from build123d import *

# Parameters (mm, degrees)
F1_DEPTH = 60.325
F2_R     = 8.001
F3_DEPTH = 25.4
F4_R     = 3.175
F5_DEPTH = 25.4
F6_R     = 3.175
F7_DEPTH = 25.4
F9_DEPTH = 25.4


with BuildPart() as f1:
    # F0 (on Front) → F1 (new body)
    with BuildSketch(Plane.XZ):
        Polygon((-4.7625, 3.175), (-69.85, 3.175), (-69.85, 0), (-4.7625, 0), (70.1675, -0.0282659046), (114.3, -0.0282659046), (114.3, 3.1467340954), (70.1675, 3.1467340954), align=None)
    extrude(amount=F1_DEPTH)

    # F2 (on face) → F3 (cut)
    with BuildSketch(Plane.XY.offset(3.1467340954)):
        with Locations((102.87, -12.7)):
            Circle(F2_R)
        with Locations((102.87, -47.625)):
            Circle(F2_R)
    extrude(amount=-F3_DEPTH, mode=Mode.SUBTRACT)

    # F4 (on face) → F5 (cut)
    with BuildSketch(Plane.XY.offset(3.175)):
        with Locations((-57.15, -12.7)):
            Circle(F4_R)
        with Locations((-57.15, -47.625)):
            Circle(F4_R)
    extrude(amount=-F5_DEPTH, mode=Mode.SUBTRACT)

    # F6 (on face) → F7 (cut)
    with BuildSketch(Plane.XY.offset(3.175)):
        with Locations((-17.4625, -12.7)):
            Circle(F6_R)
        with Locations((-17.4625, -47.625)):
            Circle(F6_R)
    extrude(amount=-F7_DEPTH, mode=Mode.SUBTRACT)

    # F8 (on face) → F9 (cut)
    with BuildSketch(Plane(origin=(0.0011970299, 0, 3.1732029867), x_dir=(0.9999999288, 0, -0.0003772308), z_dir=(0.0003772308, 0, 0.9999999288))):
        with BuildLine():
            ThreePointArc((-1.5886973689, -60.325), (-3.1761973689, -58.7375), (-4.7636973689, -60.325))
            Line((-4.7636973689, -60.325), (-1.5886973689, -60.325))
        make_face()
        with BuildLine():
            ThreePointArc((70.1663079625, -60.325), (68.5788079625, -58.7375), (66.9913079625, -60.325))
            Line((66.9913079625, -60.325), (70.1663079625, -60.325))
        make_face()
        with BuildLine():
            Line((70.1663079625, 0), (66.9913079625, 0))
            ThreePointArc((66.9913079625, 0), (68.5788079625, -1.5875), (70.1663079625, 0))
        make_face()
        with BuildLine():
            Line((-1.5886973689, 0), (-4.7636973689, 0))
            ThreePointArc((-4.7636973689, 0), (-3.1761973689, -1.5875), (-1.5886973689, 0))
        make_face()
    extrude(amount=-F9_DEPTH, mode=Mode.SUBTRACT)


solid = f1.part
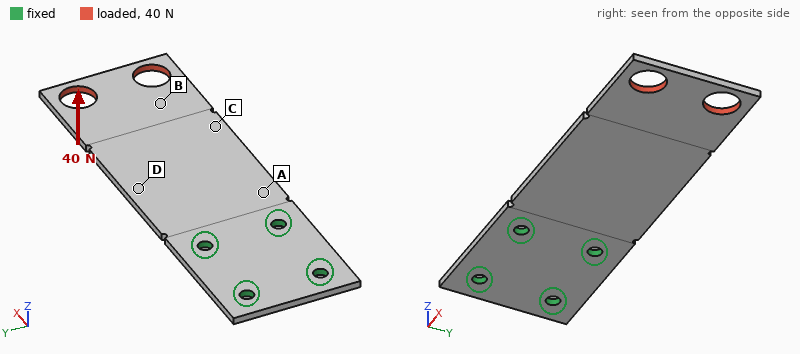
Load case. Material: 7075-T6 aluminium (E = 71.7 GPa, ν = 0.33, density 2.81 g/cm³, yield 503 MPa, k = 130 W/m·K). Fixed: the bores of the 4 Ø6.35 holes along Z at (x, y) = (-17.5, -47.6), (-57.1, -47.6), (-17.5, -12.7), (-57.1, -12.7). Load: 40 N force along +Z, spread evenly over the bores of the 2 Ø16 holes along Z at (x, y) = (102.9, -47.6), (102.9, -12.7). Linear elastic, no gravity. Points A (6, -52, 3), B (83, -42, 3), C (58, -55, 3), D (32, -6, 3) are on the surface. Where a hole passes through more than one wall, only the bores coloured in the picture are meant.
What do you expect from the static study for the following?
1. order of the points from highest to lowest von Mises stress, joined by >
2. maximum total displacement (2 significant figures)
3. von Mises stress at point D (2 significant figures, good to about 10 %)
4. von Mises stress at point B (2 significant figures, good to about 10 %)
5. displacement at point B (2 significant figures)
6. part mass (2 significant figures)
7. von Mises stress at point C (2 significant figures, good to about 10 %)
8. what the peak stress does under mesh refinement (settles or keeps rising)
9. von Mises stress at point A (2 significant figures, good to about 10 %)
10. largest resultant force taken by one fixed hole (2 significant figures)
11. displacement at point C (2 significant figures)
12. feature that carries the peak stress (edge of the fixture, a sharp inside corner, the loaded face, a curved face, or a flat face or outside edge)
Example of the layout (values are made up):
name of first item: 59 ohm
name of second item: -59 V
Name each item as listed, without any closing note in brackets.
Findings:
order of the points from highest to lowest von Mises stress, joined by >: A > D > C > B
maximum total displacement: 2.2 mm
von Mises stress at point D: 28 MPa
von Mises stress at point B: 8.5 MPa
displacement at point B: 1.5 mm
part mass: 94 g
von Mises stress at point C: 18 MPa
what the peak stress does under mesh refinement: keeps rising
von Mises stress at point A: 37 MPa
largest resultant force taken by one fixed hole: 27 N
displacement at point C: 0.88 mm
feature that carries the peak stress: edge of the fixture
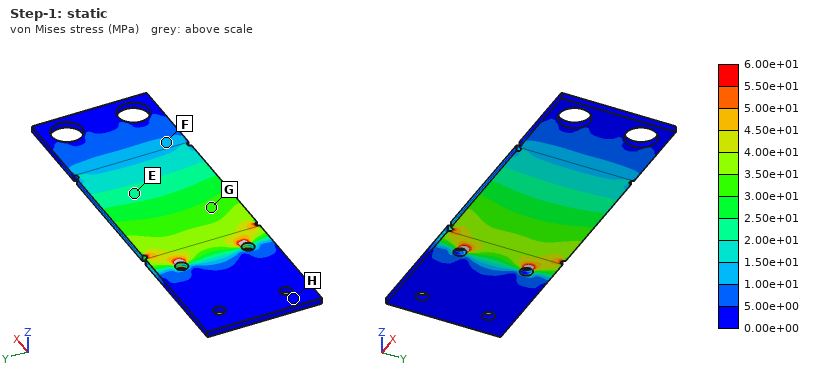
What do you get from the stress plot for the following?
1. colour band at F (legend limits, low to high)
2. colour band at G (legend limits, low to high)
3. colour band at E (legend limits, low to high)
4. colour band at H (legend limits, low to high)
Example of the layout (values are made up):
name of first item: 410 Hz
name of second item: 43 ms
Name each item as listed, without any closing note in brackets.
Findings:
colour band at F: 1.00e+01 to 1.50e+01 MPa
colour band at G: 3.00e+01 to 3.50e+01 MPa
colour band at E: 2.00e+01 to 2.50e+01 MPa
colour band at H: 0.00e+00 to 5.00e+00 MPa
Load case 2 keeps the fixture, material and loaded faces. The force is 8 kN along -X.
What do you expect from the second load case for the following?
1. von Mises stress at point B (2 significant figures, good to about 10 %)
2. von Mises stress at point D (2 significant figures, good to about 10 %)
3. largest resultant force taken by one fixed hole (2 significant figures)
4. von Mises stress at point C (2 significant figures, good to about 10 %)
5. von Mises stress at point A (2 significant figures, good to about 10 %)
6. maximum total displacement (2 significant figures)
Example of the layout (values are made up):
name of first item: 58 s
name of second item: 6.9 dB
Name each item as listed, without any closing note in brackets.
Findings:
von Mises stress at point B: 37 MPa
von Mises stress at point D: 40 MPa
largest resultant force taken by one fixed hole: 3.5 kN
von Mises stress at point C: 43 MPa
von Mises stress at point A: 42 MPa
maximum total displacement: 0.15 mm
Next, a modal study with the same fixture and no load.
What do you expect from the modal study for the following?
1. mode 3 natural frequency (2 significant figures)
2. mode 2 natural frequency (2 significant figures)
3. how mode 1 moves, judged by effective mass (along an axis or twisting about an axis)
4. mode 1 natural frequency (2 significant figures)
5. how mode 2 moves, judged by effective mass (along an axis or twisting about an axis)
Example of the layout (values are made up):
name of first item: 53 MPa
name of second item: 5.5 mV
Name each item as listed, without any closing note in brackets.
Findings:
mode 3 natural frequency: 1000 Hz
mode 2 natural frequency: 730 Hz
how mode 1 moves, judged by effective mass: along Z
mode 1 natural frequency: 170 Hz
how mode 2 moves, judged by effective mass: twisting about X
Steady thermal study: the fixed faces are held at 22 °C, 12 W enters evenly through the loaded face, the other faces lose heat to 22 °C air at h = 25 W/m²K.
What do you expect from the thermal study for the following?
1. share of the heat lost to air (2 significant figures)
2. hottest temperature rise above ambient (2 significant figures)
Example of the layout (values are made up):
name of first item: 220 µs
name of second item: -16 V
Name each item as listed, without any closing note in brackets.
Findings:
share of the heat lost to air: 56 %
hottest temperature rise above ambient: 40 K
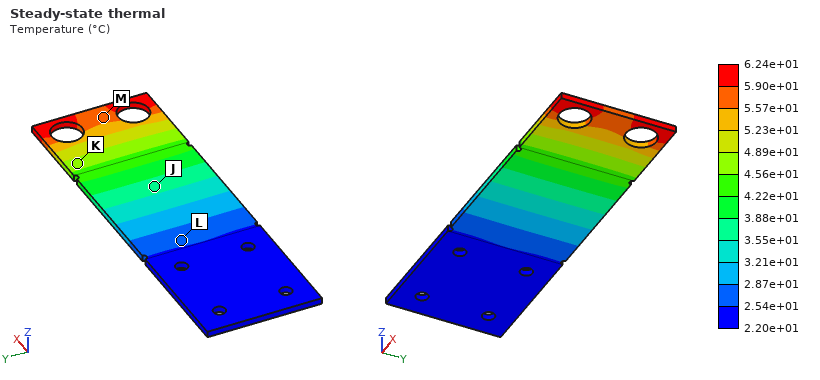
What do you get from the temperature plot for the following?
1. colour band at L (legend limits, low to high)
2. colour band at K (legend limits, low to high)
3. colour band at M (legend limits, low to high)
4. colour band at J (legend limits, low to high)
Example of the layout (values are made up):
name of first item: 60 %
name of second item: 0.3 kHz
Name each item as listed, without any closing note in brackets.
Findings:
colour band at L: 2.54e+01 to 2.87e+01 °C
colour band at K: 4.56e+01 to 4.89e+01 °C
colour band at M: 5.57e+01 to 5.90e+01 °C
colour band at J: 3.55e+01 to 3.88e+01 °C
